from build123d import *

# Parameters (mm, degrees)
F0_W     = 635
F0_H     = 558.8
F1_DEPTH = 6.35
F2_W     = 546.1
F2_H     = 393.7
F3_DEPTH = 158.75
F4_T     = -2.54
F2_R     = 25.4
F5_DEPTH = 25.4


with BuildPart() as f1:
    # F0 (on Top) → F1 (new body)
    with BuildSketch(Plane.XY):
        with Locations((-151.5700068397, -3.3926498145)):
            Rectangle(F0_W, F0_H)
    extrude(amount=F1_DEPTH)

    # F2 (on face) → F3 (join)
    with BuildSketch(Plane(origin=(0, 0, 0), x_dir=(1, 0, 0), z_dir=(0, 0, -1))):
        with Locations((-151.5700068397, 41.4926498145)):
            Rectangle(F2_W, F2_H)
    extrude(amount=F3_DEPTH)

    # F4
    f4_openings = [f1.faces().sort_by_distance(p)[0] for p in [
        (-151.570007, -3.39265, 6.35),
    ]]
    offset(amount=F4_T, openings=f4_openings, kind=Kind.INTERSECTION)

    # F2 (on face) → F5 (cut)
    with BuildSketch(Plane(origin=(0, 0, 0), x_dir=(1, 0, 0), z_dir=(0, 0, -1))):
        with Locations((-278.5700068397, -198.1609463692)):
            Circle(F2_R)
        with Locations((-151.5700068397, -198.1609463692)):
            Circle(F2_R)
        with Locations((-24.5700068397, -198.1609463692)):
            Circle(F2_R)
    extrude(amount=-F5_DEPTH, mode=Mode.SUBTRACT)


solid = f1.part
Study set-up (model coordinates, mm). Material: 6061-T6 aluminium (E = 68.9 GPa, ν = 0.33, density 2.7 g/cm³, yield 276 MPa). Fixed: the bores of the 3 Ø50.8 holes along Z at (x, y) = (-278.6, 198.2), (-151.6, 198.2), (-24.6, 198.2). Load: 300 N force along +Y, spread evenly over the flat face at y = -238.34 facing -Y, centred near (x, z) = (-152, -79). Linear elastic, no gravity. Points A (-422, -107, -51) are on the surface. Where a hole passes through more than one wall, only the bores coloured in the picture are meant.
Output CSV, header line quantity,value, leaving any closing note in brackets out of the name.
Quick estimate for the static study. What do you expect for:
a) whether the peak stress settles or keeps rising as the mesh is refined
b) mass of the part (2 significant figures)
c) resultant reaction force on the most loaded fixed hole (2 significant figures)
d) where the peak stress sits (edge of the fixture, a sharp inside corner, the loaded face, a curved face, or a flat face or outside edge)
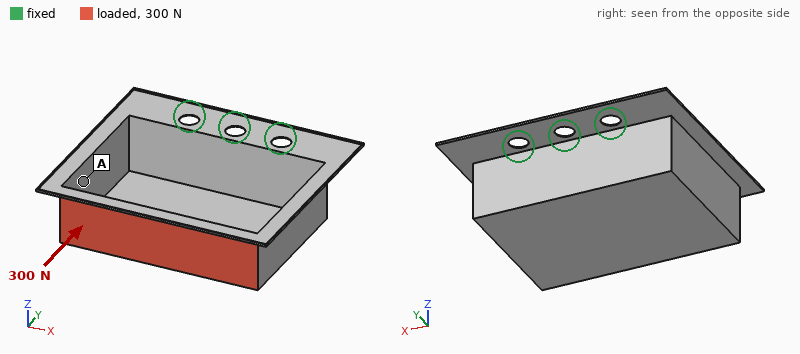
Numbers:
quantity,value
whether the peak stress settles or keeps rising as the mesh is refined,keeps rising
mass of the part,4.5 kg
resultant reaction force on the most loaded fixed hole,220 N
where the peak stress sits,edge of the fixture
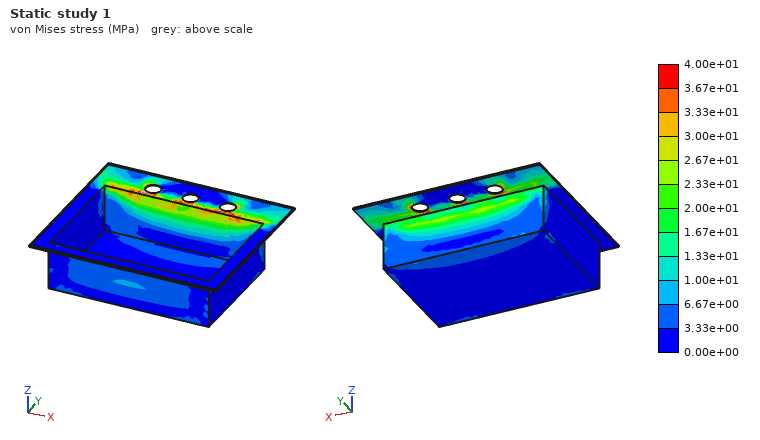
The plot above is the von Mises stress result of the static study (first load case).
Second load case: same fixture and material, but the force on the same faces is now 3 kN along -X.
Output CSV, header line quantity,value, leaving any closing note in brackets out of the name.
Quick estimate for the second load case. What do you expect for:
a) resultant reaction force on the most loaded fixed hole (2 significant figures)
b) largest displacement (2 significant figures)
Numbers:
quantity,value
resultant reaction force on the most loaded fixed hole,3.4 kN
largest displacement,6.8 mm
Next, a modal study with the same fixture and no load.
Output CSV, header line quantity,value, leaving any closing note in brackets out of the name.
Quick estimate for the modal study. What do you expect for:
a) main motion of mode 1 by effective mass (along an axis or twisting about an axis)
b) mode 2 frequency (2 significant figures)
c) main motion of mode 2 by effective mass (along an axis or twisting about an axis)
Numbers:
quantity,value
main motion of mode 1 by effective mass,along Z
mode 2 frequency,79 Hz
main motion of mode 2 by effective mass,along X
